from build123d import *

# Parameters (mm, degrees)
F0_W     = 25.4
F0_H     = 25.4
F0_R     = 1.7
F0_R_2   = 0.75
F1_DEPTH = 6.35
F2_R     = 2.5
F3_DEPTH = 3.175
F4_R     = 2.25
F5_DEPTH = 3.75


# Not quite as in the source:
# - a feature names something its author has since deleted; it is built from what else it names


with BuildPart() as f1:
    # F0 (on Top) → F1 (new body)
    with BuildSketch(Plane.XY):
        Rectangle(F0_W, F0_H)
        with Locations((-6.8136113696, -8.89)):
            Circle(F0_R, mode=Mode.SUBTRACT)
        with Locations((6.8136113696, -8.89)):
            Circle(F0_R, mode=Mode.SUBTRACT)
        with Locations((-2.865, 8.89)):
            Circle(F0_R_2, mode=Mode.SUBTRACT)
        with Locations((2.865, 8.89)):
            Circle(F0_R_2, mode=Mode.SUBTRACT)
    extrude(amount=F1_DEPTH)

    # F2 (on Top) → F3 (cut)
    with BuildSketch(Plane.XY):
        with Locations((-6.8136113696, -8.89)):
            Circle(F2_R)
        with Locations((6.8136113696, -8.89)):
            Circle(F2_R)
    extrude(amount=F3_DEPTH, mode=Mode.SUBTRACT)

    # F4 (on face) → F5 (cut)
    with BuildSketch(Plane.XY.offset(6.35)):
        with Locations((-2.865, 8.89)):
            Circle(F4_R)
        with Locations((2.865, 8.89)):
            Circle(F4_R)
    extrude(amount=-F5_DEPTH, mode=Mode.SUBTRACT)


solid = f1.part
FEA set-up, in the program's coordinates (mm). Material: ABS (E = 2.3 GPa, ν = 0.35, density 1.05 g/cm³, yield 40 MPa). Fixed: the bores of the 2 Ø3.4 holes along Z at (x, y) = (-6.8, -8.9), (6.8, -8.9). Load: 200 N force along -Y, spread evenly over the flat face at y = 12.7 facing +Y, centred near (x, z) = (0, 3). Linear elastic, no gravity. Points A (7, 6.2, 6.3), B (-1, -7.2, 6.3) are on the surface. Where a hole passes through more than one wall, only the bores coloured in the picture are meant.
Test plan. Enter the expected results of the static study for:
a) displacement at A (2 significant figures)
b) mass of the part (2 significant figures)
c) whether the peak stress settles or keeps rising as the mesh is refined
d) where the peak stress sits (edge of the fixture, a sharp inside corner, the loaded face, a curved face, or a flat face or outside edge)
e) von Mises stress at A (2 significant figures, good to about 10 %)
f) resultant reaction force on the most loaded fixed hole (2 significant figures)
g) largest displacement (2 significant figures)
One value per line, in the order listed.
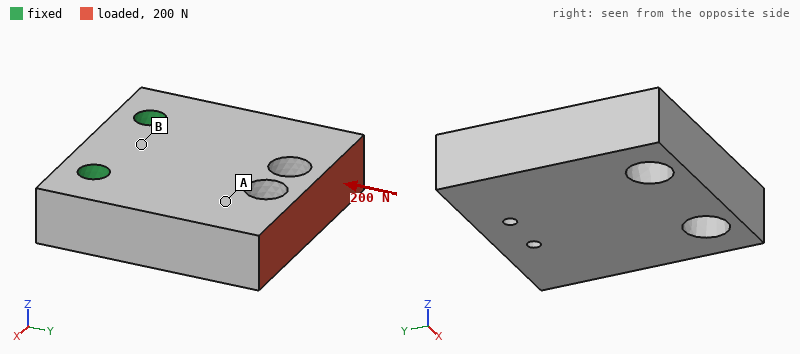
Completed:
38 µm
4.0 g
keeps rising
edge of the fixture
2.0 MPa
100 N
61 µm
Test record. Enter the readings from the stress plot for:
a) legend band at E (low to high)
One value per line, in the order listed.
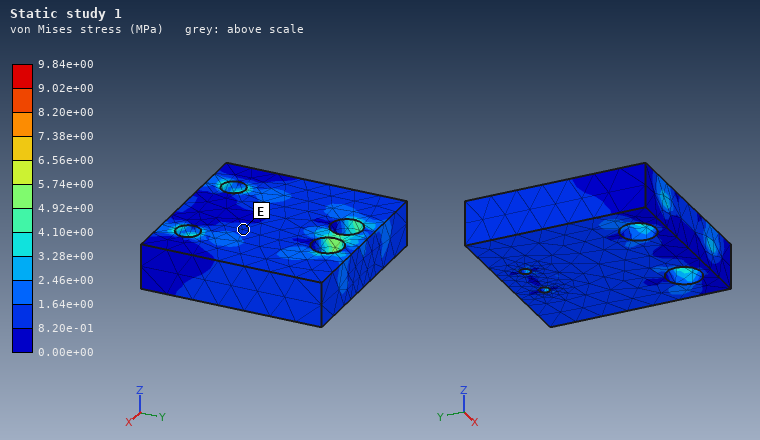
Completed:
8.20e-01 to 1.64e+00 MPa
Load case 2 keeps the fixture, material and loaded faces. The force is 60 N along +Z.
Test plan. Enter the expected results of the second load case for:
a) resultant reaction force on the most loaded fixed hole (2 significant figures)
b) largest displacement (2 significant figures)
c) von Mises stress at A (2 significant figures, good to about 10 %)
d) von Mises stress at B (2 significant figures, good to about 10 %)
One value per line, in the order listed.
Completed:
32 N
0.36 mm
3.0 MPa
4.8 MPa
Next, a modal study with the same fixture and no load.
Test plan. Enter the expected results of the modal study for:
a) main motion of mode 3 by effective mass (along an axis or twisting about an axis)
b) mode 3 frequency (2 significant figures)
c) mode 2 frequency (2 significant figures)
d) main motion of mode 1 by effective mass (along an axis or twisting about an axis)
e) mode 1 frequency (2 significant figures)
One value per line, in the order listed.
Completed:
along X
6000 Hz
4700 Hz
along Z
2100 Hz
